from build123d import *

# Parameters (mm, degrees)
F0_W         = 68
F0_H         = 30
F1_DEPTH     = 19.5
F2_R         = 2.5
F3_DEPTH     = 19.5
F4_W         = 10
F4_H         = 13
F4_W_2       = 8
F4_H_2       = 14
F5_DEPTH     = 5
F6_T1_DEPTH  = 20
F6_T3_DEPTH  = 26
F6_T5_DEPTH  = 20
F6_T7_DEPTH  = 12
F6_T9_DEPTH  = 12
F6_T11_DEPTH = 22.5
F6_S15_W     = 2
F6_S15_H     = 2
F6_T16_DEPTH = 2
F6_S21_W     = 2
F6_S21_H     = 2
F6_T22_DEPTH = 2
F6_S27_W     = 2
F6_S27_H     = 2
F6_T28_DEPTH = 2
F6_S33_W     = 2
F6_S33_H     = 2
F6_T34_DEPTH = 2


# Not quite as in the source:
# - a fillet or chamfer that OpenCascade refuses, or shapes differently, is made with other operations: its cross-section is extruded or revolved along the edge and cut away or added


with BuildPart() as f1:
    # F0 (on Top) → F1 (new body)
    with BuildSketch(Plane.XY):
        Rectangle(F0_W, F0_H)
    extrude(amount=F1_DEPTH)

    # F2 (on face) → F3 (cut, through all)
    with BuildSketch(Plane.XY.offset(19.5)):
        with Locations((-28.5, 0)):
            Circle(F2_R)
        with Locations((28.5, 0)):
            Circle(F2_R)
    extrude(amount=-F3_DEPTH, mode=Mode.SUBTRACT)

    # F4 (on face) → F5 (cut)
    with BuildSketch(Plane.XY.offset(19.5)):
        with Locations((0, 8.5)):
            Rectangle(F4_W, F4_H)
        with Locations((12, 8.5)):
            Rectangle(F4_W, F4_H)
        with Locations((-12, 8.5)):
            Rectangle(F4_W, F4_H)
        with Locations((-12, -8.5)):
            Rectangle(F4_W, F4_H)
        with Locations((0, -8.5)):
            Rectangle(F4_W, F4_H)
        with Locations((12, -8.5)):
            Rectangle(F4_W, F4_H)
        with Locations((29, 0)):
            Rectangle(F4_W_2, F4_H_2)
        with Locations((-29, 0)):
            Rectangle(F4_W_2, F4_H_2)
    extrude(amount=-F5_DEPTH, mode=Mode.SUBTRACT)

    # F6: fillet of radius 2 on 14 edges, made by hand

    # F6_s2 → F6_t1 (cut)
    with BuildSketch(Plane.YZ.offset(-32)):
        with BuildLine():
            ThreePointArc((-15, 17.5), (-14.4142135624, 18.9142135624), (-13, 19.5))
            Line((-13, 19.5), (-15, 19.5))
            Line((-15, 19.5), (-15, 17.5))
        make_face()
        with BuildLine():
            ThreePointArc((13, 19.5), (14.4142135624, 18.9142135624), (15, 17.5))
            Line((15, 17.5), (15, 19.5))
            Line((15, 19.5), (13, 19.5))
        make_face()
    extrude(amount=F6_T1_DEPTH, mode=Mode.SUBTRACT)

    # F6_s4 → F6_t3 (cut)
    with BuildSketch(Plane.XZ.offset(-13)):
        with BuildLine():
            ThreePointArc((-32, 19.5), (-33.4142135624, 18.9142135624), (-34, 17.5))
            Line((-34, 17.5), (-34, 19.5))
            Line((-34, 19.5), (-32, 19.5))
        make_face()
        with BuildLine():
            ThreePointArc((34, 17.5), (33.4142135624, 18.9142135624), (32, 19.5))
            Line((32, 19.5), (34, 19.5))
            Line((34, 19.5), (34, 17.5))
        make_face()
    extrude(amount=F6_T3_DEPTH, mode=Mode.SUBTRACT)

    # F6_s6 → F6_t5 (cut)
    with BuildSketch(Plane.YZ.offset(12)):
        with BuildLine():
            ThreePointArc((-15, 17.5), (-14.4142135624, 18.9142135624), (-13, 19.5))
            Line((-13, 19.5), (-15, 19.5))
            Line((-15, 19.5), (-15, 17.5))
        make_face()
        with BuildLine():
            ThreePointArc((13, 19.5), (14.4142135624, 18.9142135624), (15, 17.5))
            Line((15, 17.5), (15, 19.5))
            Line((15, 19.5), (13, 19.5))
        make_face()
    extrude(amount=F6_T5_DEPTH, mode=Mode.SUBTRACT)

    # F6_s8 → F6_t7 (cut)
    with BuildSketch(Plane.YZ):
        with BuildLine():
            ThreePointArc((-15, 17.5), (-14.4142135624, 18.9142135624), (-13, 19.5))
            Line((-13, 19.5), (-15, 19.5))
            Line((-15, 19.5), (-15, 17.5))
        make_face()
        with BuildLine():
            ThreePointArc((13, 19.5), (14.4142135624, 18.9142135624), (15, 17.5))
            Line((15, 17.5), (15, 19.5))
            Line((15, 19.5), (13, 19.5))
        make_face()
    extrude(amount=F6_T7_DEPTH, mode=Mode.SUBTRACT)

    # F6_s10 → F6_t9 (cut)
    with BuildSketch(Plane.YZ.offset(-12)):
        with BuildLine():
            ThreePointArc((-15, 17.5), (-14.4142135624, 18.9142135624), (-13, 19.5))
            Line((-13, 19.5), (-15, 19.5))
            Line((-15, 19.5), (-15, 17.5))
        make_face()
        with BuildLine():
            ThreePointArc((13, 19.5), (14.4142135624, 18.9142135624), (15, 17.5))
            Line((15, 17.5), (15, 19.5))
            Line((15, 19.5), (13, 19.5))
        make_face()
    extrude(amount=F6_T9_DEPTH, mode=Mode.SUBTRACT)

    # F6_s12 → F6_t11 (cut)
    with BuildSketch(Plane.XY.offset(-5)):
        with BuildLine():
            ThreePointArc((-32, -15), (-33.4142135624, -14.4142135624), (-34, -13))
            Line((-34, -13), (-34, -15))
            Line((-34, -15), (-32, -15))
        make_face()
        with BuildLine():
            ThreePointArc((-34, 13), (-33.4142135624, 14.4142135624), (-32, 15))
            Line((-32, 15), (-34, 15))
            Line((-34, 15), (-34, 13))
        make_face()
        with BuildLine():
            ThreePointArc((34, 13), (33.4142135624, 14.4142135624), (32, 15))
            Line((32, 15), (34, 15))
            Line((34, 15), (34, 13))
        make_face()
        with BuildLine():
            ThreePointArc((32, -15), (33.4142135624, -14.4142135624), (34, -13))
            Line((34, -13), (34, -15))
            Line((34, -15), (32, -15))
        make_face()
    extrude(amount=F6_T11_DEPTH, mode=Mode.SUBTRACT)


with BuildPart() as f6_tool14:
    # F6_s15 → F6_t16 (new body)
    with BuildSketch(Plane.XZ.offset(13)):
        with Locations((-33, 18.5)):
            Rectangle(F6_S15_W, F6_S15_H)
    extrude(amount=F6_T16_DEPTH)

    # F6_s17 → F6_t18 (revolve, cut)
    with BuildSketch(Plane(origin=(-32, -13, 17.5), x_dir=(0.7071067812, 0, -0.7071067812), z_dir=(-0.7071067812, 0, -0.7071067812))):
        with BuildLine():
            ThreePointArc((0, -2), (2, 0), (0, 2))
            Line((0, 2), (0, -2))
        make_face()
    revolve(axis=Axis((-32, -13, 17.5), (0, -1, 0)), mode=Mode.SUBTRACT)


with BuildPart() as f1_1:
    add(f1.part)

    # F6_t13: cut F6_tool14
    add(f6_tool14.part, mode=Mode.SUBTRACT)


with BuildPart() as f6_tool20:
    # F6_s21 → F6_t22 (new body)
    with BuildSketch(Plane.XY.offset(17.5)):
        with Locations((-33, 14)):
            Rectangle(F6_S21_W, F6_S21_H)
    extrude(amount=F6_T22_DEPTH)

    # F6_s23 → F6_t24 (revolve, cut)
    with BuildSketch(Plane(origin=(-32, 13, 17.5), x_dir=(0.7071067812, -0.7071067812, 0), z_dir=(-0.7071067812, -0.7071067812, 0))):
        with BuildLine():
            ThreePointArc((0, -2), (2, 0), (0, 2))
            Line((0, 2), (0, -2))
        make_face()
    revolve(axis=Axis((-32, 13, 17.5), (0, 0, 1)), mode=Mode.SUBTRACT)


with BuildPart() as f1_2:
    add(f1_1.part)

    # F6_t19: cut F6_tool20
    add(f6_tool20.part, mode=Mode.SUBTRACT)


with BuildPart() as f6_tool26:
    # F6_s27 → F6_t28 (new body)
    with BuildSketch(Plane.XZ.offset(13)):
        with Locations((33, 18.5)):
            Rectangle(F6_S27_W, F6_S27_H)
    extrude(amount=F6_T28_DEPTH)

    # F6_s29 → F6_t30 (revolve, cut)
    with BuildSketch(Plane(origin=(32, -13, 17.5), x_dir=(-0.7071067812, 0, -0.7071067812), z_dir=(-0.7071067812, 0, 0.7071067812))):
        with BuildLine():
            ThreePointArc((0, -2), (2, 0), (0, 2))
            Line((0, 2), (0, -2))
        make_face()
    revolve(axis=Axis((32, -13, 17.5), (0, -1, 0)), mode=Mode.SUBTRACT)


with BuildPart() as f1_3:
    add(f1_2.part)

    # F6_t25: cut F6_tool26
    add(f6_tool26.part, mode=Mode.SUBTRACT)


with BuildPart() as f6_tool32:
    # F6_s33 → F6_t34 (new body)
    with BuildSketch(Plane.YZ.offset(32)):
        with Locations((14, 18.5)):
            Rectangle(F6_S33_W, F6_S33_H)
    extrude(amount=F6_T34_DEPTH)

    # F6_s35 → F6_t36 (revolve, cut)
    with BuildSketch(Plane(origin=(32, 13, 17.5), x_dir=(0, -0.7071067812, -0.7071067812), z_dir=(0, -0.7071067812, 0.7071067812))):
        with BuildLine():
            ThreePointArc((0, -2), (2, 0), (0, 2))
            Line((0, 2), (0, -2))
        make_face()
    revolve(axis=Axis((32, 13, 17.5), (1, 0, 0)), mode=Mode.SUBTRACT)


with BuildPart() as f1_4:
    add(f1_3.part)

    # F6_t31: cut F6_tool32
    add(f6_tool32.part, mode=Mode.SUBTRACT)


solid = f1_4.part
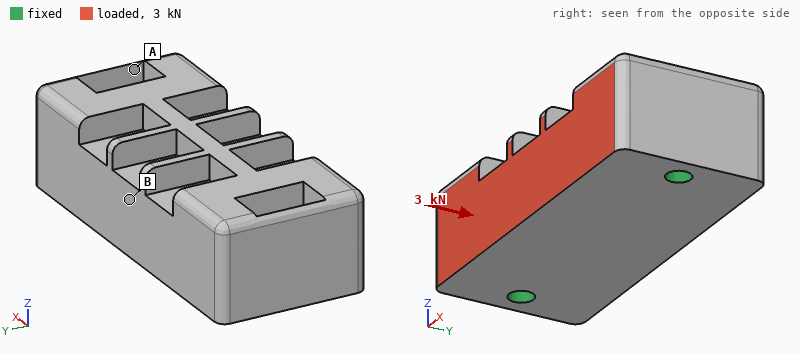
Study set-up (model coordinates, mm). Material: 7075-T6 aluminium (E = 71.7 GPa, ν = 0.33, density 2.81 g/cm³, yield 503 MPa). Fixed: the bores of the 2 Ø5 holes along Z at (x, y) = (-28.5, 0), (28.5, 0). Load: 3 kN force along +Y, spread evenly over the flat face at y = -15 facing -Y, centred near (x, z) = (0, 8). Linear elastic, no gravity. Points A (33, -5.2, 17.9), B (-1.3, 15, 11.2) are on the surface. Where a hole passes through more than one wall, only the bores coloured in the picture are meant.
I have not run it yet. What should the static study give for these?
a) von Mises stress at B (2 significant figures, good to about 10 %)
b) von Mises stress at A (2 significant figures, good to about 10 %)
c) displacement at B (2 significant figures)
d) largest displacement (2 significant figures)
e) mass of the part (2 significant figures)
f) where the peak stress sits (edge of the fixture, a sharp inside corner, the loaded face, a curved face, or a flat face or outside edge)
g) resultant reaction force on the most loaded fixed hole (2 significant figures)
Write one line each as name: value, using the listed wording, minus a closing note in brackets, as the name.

von Mises stress at B: 6.9 MPa
von Mises stress at A: 3.4 MPa
displacement at B: 3.2 µm
largest displacement: 3.9 µm
mass of the part: 96 g
where the peak stress sits: edge of the fixture
resultant reaction force on the most loaded fixed hole: 1.5 kN
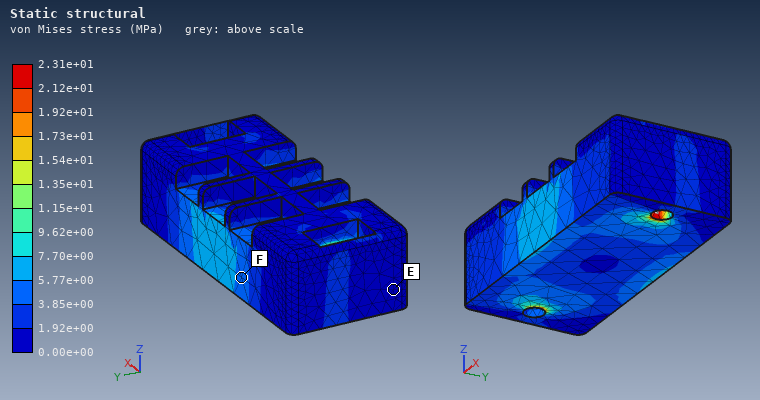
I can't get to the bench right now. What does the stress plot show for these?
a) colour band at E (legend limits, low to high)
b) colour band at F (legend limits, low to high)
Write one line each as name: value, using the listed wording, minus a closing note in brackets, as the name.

colour band at E: 0.00e+00 to 1.92e+00 MPa
colour band at F: 3.85e+00 to 5.77e+00 MPa
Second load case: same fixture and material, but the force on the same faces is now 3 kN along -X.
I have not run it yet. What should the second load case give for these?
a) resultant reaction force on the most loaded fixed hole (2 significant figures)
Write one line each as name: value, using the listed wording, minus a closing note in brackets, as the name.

resultant reaction force on the most loaded fixed hole: 1.7 kN
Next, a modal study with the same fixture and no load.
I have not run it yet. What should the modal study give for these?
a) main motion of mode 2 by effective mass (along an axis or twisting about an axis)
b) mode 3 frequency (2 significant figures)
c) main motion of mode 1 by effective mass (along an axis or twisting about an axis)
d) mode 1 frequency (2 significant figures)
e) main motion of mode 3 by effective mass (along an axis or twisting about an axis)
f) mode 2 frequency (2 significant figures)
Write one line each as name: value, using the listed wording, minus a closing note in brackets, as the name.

main motion of mode 2 by effective mass: along Y
mode 3 frequency: 17 kHz
main motion of mode 1 by effective mass: along Z
mode 1 frequency: 14 kHz
main motion of mode 3 by effective mass: along Y
mode 2 frequency: 16 kHz
